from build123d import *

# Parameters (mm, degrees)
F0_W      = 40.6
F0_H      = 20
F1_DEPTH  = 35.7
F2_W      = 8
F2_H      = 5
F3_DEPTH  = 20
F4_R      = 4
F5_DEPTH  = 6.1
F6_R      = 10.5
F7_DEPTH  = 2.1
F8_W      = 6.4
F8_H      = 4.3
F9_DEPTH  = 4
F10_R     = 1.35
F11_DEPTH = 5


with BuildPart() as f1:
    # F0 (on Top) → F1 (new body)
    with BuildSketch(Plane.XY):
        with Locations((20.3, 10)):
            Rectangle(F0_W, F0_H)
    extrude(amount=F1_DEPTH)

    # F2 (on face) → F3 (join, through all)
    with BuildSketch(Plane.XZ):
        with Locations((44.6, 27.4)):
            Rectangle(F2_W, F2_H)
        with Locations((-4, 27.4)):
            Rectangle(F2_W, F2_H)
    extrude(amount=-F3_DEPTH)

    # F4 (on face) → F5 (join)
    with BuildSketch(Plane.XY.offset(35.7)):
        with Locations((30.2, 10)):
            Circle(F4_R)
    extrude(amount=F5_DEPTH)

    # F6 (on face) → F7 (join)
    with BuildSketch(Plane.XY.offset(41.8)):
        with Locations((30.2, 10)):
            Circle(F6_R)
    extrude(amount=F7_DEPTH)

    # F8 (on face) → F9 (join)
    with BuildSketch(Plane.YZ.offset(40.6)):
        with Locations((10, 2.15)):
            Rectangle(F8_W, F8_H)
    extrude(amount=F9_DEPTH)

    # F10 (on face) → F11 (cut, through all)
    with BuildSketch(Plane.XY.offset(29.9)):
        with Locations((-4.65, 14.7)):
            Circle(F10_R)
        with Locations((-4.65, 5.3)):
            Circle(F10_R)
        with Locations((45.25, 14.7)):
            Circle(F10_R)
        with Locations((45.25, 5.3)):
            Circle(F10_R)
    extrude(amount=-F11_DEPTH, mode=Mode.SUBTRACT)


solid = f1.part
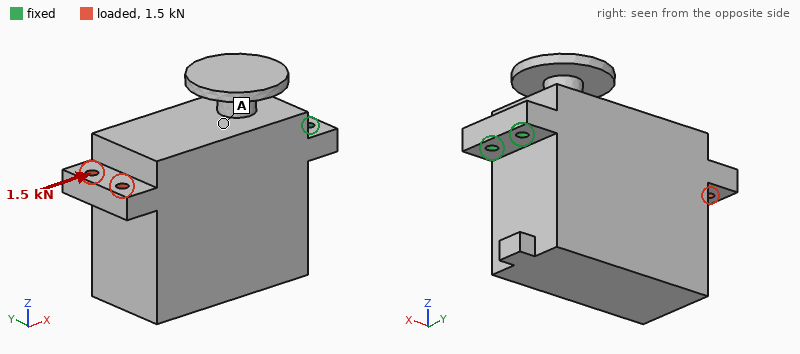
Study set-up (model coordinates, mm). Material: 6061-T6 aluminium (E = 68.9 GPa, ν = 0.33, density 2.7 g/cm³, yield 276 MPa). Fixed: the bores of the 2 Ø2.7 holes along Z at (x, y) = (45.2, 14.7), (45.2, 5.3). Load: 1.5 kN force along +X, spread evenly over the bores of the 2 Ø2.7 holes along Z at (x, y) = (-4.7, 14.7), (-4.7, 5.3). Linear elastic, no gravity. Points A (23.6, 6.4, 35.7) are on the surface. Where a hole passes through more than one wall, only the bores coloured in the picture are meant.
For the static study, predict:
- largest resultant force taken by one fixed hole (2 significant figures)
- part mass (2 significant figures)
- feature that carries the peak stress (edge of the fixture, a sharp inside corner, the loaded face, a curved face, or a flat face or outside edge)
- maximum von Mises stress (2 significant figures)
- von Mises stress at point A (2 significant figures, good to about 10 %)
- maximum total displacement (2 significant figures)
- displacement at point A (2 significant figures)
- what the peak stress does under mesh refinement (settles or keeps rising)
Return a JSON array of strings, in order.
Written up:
["750 N", "85 g", "the loaded face", "47 MPa", "5.4 MPa", "7.5 µm", "3.0 µm", "settles"]
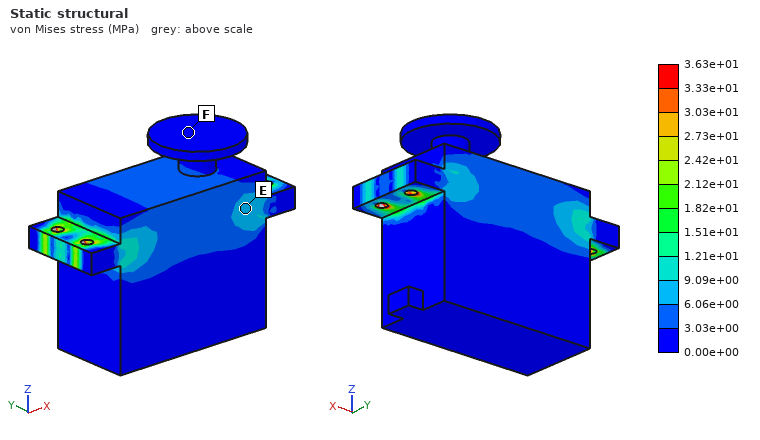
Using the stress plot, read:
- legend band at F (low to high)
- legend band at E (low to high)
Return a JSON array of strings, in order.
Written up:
["0.00e+00 to 3.03e+00 MPa", "6.06e+00 to 9.09e+00 MPa"]
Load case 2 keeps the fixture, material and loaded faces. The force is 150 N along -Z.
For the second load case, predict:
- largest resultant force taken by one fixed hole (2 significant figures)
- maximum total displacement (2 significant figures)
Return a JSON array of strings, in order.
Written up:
["75 N", "0.16 mm"]
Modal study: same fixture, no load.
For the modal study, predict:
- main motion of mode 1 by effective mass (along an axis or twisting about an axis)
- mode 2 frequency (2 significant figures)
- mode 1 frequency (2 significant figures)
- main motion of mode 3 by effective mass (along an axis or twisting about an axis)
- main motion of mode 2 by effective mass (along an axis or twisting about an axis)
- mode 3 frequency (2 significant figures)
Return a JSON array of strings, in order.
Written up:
["along Z", "2400 Hz", "900 Hz", "twisting about X", "along Y", "4200 Hz"]
